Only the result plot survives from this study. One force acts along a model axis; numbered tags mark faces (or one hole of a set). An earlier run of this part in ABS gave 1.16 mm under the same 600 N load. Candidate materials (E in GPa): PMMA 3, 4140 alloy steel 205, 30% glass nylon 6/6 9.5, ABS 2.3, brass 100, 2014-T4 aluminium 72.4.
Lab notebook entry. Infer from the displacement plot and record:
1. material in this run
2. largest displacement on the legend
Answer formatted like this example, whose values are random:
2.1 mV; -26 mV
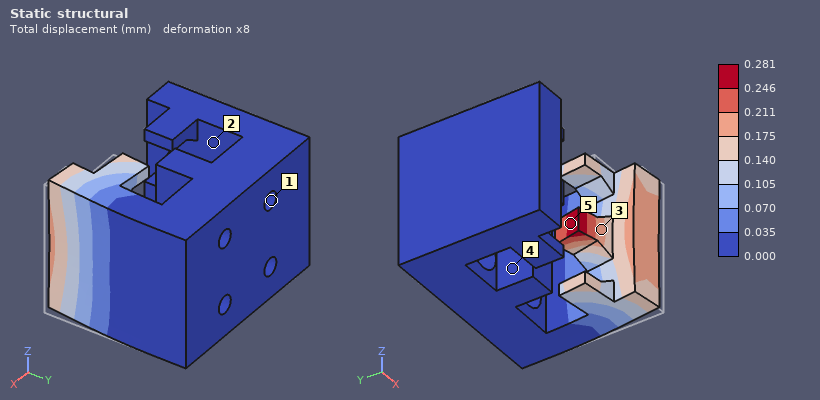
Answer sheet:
30% glass nylon 6/6; 0.281 mm
